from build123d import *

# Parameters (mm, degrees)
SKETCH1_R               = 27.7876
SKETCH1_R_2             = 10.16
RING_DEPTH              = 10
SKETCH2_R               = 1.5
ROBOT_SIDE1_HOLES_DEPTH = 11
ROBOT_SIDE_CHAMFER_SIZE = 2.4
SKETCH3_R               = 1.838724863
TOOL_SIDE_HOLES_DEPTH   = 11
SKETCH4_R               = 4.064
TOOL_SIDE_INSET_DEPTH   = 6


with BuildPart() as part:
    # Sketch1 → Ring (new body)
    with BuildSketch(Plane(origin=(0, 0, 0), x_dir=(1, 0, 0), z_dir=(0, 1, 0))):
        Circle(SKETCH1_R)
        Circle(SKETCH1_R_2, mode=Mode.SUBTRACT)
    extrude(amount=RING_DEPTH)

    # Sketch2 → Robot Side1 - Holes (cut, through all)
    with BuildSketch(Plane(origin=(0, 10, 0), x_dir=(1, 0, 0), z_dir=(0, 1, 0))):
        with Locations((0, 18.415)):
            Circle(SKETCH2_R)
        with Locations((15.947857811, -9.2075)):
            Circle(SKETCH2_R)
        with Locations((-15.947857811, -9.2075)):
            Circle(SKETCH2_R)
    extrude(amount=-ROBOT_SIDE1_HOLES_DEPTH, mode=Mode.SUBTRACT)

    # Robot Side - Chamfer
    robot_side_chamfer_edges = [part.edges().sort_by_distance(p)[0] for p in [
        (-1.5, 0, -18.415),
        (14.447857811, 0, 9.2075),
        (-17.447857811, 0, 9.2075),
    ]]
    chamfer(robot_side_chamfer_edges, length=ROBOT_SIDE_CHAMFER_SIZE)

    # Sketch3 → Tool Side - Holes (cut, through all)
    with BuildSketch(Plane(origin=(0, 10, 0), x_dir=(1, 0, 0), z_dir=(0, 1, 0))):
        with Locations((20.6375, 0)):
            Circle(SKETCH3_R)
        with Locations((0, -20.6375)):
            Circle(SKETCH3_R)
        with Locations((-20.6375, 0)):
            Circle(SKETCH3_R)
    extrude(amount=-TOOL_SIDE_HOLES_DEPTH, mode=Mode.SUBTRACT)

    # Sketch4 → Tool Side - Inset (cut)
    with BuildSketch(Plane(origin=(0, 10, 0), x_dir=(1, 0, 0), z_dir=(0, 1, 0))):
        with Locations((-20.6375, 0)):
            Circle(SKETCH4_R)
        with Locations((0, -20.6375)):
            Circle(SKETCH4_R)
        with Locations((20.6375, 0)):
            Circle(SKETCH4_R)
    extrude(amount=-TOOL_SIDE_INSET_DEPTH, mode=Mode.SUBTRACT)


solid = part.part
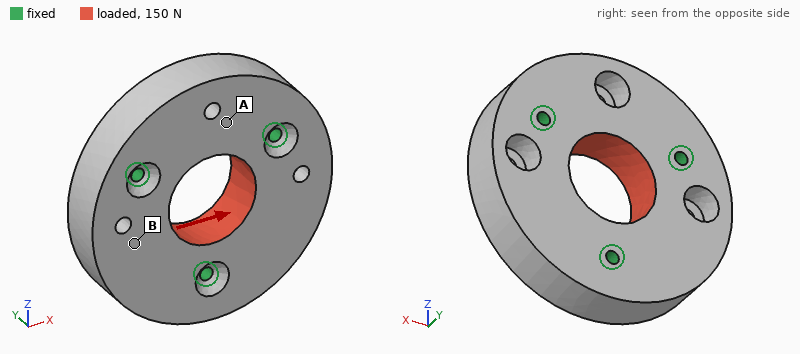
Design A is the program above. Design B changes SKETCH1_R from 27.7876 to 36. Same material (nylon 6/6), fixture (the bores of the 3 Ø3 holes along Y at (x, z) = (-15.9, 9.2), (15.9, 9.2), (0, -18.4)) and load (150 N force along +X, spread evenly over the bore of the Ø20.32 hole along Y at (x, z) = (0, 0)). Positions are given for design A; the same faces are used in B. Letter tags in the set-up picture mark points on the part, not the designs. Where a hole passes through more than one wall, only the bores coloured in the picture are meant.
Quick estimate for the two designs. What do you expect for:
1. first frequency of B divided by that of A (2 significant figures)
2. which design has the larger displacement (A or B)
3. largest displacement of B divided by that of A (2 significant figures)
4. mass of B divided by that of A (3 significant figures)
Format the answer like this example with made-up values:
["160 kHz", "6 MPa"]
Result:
["0.59", "A", "0.85", "1.84"]
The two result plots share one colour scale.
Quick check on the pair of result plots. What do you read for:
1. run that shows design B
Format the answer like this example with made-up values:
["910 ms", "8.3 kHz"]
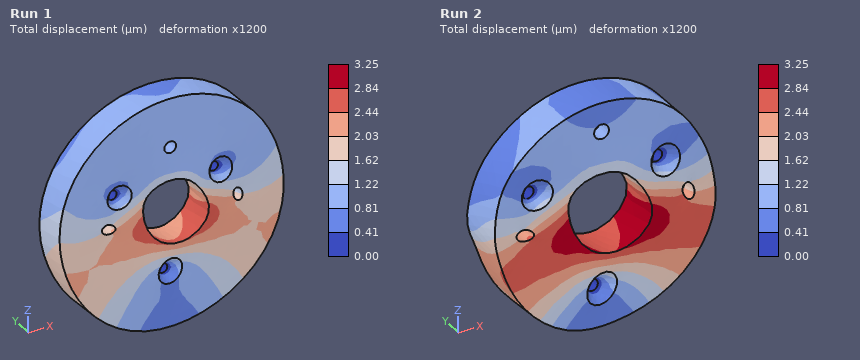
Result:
["Run 1"]
